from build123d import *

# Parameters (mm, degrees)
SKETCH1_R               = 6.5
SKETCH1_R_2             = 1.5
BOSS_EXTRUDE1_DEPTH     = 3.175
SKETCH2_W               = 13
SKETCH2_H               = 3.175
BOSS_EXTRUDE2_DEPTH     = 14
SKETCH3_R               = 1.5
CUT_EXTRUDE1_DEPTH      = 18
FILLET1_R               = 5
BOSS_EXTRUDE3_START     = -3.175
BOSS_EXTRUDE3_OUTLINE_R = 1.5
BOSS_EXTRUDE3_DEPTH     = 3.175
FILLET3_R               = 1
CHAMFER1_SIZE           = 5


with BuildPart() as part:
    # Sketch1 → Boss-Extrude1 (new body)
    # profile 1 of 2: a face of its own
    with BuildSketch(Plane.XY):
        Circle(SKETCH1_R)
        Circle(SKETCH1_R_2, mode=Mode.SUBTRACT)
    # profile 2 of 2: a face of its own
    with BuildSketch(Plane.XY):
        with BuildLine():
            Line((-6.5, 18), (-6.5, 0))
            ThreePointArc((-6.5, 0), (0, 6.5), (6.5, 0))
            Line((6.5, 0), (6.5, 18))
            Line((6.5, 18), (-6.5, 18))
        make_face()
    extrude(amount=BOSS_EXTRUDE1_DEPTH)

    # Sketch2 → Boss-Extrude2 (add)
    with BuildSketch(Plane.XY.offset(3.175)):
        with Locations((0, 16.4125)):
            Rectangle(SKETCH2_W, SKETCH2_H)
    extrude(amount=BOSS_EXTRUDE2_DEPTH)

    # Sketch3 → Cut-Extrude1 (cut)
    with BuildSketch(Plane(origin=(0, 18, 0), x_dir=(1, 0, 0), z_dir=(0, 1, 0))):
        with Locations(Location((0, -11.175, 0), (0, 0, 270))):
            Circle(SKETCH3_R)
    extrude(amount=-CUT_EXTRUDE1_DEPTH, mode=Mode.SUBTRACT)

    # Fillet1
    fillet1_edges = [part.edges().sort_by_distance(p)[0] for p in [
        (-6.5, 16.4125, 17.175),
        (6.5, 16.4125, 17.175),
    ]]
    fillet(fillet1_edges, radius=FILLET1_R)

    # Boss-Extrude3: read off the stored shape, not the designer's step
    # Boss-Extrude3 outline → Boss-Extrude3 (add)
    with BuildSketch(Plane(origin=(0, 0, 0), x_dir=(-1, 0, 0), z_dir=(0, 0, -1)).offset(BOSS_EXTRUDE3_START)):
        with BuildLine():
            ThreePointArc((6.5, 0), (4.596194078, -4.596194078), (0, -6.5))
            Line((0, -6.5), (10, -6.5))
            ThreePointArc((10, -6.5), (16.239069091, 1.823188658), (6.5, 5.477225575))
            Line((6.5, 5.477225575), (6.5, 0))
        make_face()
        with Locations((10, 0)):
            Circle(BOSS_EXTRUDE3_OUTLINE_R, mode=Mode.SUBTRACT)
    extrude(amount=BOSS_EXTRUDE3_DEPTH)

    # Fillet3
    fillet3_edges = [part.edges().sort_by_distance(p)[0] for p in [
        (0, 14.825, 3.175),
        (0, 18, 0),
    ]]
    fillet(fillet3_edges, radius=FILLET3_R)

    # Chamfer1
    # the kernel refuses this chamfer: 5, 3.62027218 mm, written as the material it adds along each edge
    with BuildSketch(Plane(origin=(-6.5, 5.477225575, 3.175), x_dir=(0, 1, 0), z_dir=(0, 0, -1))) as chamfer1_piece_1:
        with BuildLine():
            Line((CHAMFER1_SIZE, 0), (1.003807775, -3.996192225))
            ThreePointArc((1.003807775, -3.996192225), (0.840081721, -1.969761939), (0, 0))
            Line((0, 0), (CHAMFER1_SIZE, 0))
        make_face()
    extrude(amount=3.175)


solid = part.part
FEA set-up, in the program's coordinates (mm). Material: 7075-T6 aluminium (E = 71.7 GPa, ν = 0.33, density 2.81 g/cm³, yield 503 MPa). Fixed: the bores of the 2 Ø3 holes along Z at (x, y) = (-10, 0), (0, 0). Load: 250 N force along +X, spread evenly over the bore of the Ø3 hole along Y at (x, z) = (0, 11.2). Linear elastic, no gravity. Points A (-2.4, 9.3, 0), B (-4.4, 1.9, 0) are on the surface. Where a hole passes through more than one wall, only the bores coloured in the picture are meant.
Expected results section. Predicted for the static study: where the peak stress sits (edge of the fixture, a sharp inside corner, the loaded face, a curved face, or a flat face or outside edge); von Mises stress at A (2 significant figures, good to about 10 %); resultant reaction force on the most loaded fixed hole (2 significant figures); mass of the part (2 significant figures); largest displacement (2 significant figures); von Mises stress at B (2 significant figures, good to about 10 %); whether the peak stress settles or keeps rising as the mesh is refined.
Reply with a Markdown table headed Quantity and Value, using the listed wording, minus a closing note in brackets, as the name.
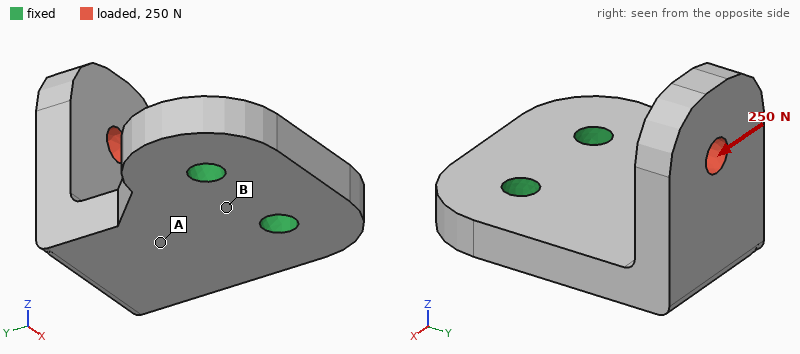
| Quantity | Value |
|---|---|
| where the peak stress sits | edge of the fixture |
| von Mises stress at A | 75 MPa |
| resultant reaction force on the most loaded fixed hole | 410 N |
| mass of the part | 5.2 g |
| largest displacement | 0.13 mm |
| von Mises stress at B | 24 MPa |
| whether the peak stress settles or keeps rising as the mesh is refined | keeps rising |
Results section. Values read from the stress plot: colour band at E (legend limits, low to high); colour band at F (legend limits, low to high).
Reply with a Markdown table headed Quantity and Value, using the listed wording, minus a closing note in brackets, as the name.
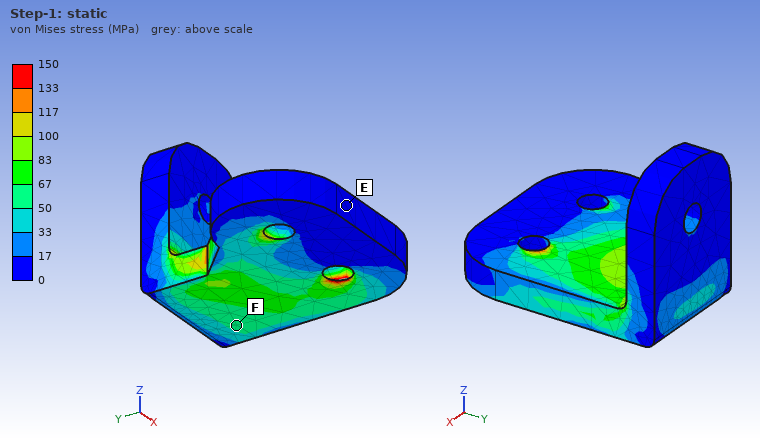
| Quantity | Value |
|---|---|
| colour band at E | 0 to 17 MPa |
| colour band at F | 50 to 67 MPa |
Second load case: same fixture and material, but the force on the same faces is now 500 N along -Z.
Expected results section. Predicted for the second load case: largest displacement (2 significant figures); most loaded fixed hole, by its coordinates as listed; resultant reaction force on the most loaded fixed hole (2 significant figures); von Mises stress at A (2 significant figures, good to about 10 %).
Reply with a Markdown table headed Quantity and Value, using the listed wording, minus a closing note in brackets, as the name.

| Quantity | Value |
|---|---|
| largest displacement | 0.42 mm |
| most loaded fixed hole, by its coordinates as listed | (0, 0) |
| resultant reaction force on the most loaded fixed hole | 440 N |
| von Mises stress at A | 150 MPa |
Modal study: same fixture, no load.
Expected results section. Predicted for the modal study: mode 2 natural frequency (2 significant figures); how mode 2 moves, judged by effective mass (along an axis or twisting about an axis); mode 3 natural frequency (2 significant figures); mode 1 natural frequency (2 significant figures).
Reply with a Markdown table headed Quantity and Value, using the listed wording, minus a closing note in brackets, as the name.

| Quantity | Value |
|---|---|
| mode 2 natural frequency | 7000 Hz |
| how mode 2 moves, judged by effective mass | along X |
| mode 3 natural frequency | 11 kHz |
| mode 1 natural frequency | 4000 Hz |
